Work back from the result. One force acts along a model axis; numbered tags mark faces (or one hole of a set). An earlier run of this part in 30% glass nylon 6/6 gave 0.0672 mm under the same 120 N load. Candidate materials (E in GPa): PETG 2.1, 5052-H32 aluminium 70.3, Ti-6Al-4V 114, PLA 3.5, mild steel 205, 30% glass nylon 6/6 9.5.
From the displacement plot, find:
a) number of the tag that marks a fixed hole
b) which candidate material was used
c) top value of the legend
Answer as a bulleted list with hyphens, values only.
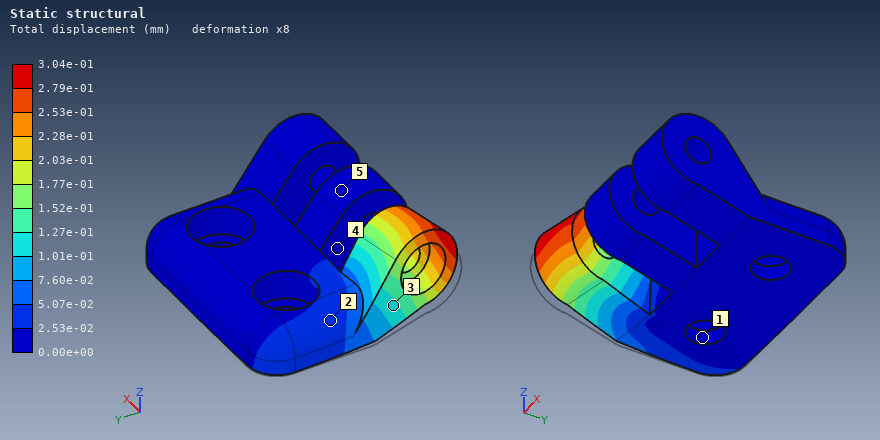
- 1
- PETG
- 3.04e-01 mm
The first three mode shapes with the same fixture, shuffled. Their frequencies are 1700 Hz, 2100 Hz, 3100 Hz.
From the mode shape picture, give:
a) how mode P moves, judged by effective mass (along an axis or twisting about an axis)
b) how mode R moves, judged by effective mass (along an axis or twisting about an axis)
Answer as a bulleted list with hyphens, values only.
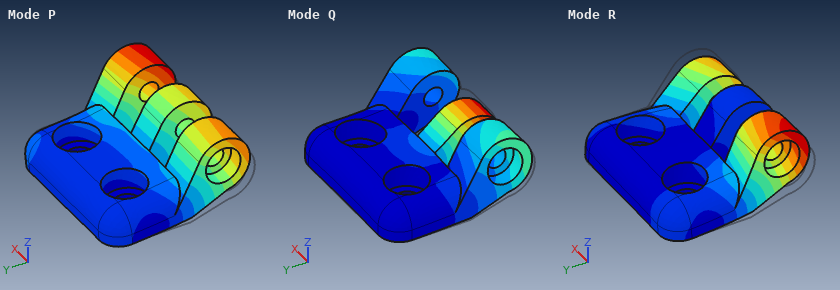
- along Z
- twisting about Y
